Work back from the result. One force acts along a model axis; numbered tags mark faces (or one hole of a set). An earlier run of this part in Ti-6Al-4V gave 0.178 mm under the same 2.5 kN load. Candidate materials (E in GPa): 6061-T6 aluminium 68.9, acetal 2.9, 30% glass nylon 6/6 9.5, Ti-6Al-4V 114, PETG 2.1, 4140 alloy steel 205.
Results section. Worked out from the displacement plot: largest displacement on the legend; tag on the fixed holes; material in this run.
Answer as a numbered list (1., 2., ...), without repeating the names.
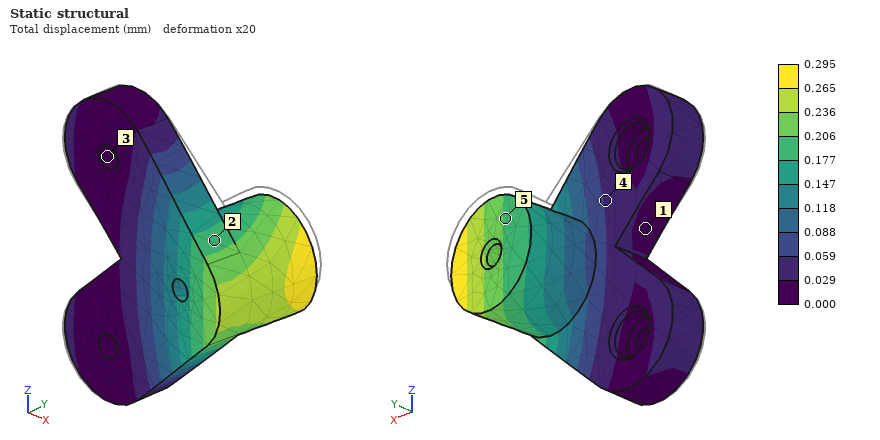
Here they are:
1. 0.295 mm
2. 3
3. 6061-T6 aluminium
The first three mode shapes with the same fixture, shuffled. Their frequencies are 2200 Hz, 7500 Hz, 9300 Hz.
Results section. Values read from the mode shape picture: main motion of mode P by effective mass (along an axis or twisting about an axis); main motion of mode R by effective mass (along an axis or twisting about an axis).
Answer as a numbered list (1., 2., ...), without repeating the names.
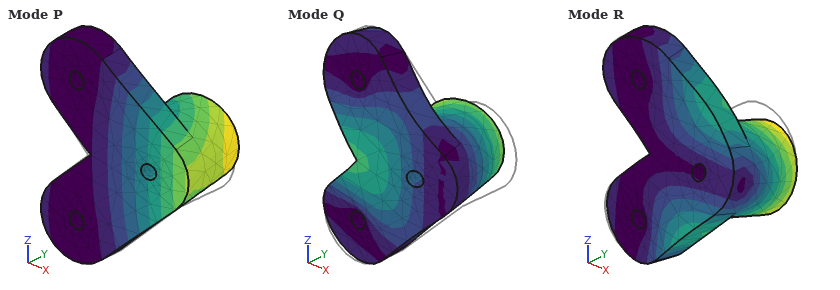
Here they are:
1. along Y
2. along Z
